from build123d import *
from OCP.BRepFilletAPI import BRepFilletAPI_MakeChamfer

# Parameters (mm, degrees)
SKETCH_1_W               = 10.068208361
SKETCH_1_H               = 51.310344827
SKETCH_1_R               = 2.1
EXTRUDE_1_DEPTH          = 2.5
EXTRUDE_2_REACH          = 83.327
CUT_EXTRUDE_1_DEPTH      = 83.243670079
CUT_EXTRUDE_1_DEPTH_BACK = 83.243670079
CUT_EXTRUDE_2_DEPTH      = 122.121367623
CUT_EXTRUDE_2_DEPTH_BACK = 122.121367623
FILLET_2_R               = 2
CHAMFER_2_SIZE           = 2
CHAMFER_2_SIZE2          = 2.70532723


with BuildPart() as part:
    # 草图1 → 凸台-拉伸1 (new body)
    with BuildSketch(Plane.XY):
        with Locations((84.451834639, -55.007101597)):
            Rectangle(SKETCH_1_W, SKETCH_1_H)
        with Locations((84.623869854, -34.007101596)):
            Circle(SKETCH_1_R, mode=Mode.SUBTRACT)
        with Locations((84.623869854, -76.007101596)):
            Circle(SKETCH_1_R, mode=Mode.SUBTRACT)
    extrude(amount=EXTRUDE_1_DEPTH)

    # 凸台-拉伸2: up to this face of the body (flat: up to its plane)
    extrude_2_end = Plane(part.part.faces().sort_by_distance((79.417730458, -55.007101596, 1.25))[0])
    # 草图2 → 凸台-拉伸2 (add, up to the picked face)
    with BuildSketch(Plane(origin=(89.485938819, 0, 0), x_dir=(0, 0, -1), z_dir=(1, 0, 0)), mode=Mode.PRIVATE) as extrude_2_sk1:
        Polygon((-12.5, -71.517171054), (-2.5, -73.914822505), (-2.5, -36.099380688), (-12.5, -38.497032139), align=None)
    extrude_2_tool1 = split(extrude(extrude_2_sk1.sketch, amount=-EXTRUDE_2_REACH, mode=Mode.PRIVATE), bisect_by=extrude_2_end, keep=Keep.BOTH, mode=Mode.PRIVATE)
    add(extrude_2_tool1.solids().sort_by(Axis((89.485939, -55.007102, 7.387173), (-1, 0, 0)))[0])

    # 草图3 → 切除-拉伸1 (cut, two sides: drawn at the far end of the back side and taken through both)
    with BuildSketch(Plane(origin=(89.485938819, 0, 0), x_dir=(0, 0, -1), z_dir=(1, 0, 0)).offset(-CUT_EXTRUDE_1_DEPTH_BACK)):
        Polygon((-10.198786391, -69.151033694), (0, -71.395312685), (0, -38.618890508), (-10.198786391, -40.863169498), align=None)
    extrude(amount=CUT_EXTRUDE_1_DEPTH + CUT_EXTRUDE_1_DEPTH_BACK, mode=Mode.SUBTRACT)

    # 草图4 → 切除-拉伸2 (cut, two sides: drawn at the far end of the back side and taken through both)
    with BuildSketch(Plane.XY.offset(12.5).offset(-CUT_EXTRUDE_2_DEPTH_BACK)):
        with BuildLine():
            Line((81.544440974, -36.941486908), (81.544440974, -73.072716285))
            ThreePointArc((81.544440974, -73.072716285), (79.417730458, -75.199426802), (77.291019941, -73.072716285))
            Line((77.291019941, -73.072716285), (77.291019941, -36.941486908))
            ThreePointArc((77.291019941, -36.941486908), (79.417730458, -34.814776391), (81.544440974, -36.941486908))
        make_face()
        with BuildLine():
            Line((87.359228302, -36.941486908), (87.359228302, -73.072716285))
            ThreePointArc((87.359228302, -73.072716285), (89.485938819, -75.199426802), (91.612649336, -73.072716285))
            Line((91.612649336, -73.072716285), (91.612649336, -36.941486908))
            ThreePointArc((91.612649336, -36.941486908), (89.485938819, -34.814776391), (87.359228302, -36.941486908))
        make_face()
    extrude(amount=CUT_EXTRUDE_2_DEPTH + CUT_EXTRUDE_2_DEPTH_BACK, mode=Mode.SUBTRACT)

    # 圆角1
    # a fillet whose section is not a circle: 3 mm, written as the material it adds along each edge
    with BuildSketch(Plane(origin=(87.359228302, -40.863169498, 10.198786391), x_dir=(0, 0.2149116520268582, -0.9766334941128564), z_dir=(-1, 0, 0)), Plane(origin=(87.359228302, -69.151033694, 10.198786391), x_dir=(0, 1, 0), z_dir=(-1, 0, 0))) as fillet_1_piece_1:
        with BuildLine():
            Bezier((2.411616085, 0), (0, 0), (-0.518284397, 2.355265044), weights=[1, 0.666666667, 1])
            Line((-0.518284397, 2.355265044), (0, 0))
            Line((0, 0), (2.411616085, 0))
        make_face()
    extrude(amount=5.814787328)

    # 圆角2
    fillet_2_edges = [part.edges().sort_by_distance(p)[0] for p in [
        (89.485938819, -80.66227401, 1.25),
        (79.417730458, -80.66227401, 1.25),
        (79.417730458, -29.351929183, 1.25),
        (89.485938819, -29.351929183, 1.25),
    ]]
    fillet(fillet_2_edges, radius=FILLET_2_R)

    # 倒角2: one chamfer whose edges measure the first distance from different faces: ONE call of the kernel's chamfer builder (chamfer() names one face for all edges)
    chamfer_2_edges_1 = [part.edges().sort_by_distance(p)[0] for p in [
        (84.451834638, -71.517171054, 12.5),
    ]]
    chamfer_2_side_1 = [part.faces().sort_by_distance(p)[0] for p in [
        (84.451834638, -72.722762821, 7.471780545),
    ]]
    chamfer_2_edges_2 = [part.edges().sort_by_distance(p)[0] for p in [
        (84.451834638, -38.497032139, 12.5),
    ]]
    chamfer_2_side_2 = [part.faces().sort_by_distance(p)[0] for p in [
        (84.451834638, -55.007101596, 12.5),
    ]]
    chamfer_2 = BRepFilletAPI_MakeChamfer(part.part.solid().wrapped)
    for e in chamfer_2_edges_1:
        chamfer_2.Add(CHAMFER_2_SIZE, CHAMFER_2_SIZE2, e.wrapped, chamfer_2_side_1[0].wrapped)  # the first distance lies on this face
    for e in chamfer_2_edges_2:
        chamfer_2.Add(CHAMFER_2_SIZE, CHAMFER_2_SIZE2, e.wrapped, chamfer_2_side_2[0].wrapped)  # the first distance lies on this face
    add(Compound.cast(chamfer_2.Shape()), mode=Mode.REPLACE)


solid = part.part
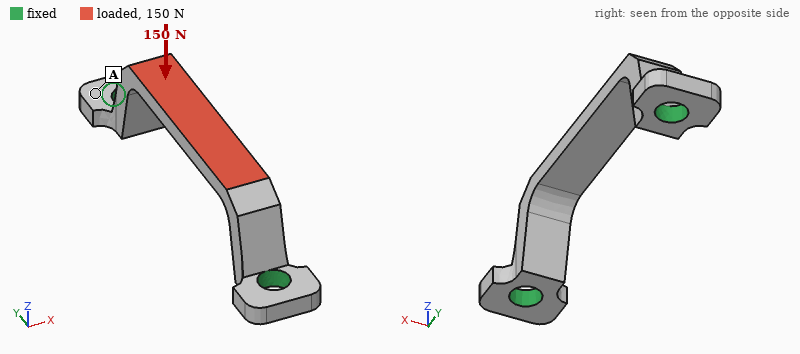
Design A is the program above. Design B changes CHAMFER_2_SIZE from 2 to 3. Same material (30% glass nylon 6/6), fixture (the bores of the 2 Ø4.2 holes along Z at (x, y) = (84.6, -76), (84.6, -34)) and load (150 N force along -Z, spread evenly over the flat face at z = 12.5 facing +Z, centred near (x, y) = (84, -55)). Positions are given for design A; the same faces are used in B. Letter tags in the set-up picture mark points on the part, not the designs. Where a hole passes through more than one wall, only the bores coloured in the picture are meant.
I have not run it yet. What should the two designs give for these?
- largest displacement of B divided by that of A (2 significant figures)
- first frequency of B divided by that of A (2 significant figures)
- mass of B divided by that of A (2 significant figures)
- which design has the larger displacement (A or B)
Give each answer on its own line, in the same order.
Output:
1.1
1.0
0.99
B
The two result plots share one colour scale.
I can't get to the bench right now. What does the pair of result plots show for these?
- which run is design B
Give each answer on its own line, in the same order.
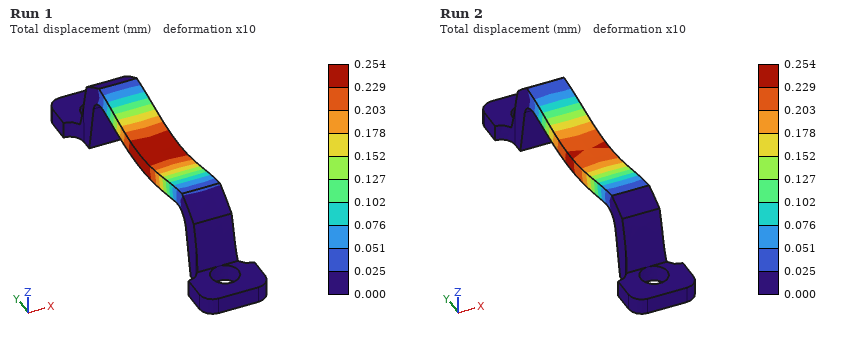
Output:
Run 1
